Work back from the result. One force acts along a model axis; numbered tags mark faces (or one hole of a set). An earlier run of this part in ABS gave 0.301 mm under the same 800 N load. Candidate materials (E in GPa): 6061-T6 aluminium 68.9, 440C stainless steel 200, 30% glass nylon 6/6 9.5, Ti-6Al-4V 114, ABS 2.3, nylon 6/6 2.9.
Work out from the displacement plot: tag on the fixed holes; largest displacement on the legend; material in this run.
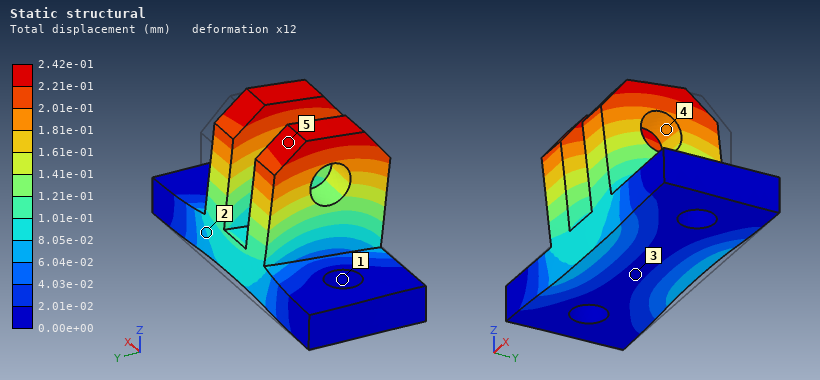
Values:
1
2.42e-01 mm
nylon 6/6
